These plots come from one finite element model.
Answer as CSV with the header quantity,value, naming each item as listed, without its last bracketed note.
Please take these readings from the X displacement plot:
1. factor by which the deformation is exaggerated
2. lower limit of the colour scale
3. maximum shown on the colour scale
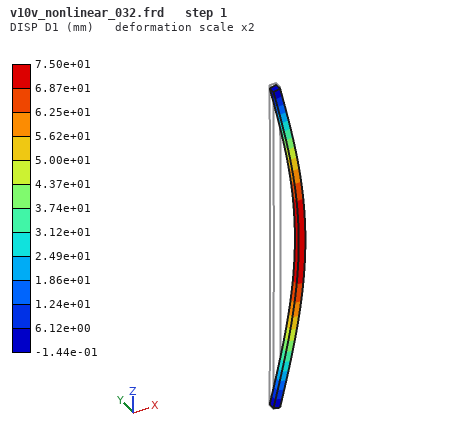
quantity,value
factor by which the deformation is exaggerated,2
lower limit of the colour scale,-1.44e-01 mm
maximum shown on the colour scale,7.50e+01 mm
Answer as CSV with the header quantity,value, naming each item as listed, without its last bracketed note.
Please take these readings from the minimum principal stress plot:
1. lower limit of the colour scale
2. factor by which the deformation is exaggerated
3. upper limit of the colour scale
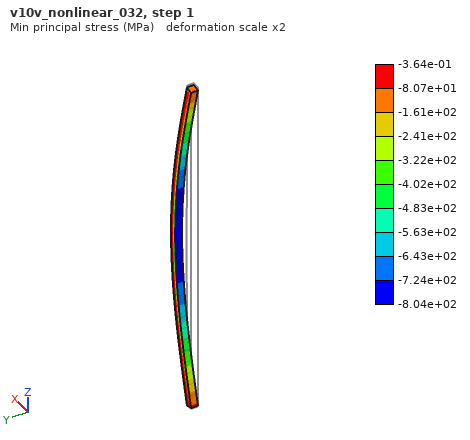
quantity,value
lower limit of the colour scale,-8.04e+02 MPa
factor by which the deformation is exaggerated,2
upper limit of the colour scale,-3.64e-01 MPa
